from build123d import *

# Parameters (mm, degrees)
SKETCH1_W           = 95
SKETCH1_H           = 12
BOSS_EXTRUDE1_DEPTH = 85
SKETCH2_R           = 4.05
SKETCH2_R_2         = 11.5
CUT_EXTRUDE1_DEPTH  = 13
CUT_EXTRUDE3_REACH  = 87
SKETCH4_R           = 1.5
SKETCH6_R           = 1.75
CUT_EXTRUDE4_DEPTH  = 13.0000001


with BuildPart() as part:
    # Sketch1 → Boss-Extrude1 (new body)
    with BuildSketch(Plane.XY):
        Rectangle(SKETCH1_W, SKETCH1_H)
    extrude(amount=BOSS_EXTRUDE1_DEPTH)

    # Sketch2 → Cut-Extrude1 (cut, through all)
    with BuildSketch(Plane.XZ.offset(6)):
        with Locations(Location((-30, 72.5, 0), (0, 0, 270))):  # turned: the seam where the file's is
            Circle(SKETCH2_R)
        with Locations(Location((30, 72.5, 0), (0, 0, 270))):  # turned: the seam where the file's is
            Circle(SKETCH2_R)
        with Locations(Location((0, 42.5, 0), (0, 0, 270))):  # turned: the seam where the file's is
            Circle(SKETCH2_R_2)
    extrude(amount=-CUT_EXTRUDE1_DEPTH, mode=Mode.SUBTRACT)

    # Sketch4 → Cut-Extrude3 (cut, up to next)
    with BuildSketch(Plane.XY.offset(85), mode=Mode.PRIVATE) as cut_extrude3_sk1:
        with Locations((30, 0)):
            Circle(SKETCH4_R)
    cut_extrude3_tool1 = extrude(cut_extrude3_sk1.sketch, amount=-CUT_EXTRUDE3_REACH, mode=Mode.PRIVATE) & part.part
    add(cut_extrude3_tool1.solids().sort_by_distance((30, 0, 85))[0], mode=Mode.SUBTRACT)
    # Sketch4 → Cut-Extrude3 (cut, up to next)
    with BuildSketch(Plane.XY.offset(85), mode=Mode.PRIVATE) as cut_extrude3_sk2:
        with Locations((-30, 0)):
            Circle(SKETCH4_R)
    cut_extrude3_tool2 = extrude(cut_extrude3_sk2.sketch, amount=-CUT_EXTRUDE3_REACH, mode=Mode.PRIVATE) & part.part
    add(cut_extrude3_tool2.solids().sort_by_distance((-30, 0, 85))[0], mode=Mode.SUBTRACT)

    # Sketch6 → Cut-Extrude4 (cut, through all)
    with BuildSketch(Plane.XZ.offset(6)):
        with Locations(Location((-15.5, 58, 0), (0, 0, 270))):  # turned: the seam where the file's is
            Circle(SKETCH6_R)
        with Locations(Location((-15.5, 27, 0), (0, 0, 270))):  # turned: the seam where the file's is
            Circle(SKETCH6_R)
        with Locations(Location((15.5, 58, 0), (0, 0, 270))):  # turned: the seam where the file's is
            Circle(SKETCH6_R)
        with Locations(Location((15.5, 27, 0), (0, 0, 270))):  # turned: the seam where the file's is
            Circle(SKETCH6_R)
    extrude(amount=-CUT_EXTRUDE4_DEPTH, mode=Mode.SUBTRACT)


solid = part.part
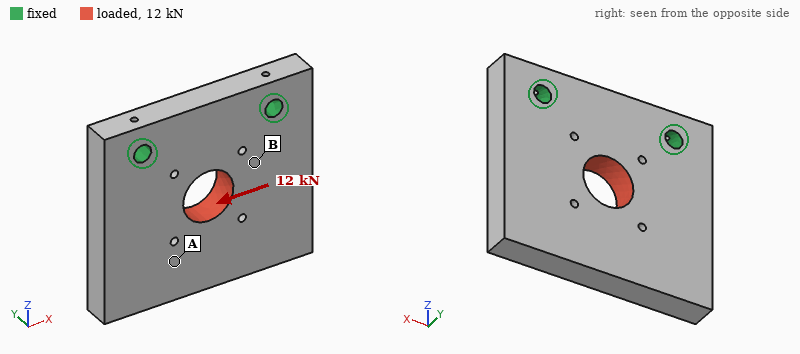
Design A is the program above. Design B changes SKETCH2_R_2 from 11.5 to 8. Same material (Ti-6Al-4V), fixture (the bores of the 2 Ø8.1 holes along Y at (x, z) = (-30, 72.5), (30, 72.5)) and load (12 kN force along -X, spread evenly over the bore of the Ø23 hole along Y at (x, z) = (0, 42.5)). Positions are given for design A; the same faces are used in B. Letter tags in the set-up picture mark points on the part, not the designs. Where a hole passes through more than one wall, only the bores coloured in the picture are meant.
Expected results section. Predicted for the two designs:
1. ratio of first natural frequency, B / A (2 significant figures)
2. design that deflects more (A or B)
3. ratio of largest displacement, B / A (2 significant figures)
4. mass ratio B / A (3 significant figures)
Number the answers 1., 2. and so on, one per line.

1. 1.0
2. A
3. 0.86
4. 1.03
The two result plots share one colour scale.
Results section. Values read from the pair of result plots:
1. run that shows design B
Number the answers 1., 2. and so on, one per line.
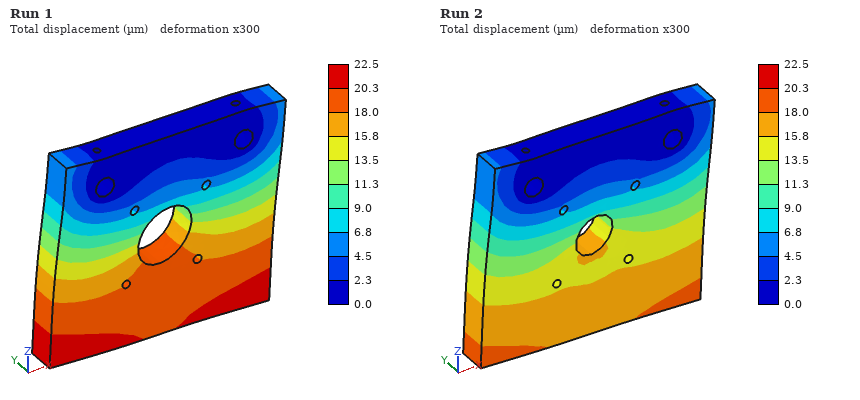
1. Run 2
